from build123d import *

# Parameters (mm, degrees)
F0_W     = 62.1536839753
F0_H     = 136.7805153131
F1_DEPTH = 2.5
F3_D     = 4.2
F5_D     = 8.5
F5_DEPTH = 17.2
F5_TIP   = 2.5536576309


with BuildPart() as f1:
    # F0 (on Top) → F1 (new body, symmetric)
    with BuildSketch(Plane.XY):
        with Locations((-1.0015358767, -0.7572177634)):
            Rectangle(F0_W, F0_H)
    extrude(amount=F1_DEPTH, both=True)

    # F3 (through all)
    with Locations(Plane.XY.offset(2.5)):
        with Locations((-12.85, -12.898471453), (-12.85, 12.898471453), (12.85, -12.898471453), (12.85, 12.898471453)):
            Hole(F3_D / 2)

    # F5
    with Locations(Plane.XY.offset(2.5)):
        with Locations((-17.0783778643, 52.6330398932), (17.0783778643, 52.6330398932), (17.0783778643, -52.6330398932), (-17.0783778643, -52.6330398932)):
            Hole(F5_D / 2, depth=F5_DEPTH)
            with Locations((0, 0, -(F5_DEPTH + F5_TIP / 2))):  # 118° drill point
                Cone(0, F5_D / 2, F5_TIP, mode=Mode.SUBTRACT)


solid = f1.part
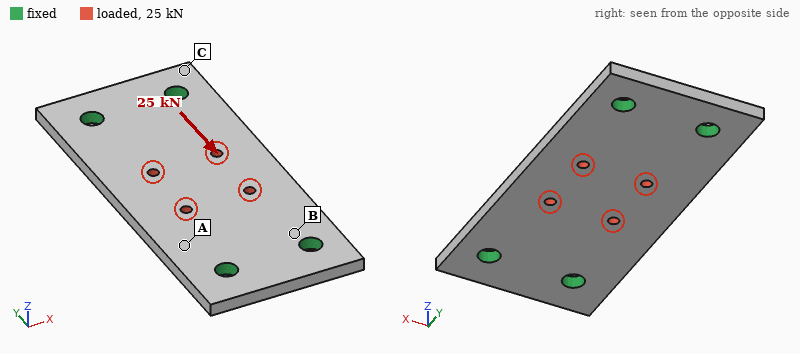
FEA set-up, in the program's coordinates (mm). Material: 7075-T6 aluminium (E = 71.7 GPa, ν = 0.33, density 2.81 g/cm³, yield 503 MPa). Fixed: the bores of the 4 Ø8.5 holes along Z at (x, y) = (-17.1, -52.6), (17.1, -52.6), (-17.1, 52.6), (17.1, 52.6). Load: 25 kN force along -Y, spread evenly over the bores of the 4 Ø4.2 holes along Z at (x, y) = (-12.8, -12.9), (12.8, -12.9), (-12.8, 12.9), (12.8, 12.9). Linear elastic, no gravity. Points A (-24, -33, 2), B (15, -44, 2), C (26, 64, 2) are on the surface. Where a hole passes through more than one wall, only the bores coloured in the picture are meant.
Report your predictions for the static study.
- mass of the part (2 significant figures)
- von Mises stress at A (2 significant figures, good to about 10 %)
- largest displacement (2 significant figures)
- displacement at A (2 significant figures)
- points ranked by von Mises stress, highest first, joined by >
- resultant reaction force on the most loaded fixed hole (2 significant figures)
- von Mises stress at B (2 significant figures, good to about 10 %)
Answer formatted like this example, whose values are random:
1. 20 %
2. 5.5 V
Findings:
1. 120 g
2. 36 MPa
3. 33 µm
4. 14 µm
5. B > A > C
6. 6.4 kN
7. 68 MPa
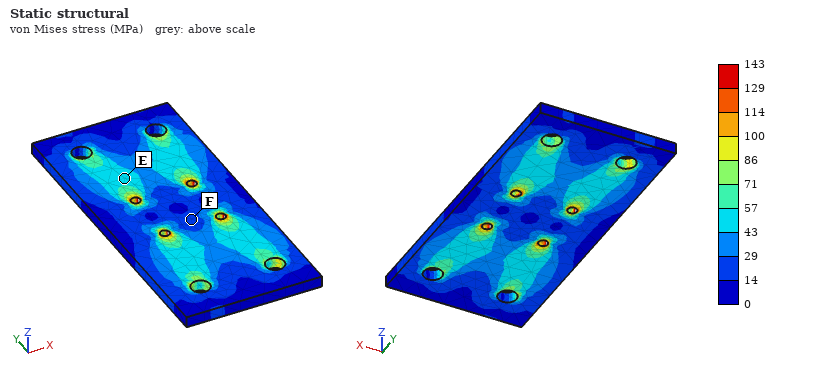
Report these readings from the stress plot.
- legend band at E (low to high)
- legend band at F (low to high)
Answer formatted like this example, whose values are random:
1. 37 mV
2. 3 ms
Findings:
1. 43 to 57 MPa
2. 14 to 29 MPa
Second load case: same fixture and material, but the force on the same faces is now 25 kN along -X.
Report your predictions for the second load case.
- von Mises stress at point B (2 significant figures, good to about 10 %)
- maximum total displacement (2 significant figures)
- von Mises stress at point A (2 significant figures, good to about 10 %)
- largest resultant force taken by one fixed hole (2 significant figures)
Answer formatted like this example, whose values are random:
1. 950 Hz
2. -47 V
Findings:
1. 100 MPa
2. 97 µm
3. 47 MPa
4. 9.1 kN
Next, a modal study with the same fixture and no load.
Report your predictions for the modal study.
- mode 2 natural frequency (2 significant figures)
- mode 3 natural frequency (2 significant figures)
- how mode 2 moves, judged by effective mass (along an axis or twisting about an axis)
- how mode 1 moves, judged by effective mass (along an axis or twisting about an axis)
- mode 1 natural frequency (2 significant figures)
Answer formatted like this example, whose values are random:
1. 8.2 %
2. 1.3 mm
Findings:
1. 3500 Hz
2. 6700 Hz
3. twisting about Y
4. along Z
5. 2500 Hz
